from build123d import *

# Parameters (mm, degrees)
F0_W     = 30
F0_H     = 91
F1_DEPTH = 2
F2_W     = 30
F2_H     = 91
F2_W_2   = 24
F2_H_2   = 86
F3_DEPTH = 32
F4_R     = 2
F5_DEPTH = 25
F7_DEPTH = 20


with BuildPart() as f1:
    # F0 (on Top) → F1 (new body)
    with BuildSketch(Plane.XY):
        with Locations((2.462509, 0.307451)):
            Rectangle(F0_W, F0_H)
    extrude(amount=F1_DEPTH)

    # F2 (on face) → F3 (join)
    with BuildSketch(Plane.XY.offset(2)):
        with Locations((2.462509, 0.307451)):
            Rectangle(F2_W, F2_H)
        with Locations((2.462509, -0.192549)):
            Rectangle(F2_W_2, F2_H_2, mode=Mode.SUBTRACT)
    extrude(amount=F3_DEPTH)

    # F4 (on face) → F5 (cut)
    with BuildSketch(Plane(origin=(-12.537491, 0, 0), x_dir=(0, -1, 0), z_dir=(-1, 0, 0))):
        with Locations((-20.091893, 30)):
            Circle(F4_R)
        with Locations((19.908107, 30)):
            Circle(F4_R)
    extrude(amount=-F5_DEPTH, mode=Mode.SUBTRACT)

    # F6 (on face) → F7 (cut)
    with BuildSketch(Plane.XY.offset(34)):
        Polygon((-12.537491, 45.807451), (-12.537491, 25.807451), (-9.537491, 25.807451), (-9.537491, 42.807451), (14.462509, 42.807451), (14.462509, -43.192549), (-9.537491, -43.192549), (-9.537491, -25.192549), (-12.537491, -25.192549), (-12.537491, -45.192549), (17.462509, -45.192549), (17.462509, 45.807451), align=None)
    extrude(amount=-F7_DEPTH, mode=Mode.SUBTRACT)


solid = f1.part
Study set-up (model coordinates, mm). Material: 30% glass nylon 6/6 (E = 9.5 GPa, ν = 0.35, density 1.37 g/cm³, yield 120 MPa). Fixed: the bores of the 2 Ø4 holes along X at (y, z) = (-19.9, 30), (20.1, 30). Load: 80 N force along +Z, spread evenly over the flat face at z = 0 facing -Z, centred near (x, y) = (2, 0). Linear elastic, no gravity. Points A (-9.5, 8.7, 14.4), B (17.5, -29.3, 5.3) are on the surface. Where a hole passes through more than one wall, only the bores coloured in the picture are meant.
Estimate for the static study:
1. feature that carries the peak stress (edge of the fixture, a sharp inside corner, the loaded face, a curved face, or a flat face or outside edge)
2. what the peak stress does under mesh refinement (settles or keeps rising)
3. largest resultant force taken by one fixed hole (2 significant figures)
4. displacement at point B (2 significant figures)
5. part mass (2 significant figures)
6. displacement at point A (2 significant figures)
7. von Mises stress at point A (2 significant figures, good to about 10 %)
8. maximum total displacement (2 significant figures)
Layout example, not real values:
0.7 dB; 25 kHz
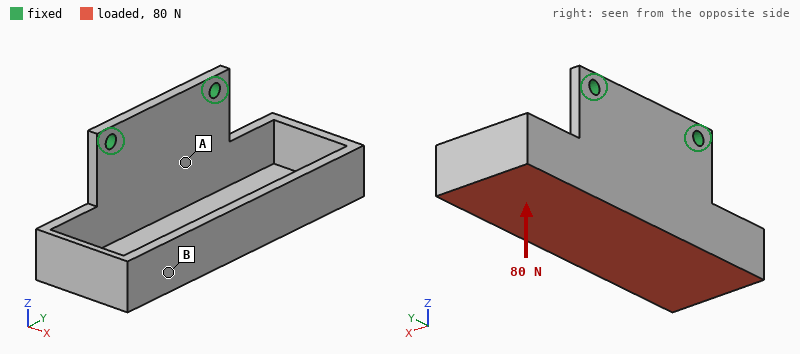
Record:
edge of the fixture; keeps rising; 41 N; 1.1 mm; 23 g; 0.18 mm; 11 MPa; 1.1 mm
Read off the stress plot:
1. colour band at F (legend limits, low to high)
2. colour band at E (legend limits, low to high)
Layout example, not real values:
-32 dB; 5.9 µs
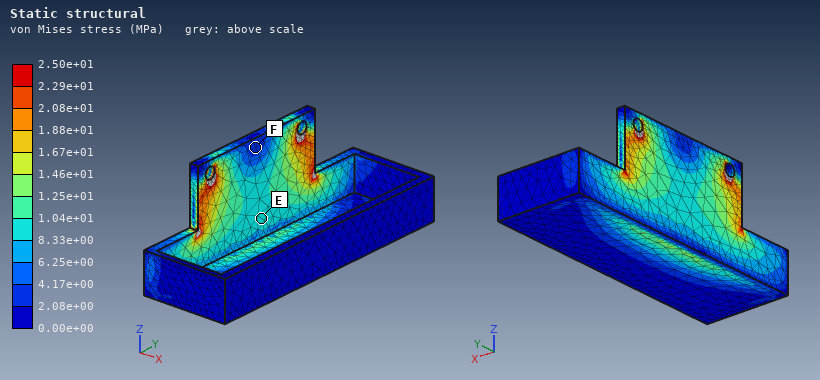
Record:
2.08e+00 to 4.17e+00 MPa; 8.33e+00 to 1.04e+01 MPa
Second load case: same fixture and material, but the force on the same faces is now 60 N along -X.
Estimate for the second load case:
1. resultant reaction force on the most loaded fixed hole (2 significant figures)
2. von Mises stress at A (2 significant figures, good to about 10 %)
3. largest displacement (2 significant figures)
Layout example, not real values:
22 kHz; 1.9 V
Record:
30 N; 9.5 MPa; 1.0 mm
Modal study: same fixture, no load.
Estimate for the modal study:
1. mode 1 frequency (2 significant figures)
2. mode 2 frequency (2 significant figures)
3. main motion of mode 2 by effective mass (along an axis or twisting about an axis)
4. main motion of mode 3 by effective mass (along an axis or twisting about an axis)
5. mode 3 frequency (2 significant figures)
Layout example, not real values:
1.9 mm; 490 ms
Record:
310 Hz; 430 Hz; along Y; along X; 770 Hz
